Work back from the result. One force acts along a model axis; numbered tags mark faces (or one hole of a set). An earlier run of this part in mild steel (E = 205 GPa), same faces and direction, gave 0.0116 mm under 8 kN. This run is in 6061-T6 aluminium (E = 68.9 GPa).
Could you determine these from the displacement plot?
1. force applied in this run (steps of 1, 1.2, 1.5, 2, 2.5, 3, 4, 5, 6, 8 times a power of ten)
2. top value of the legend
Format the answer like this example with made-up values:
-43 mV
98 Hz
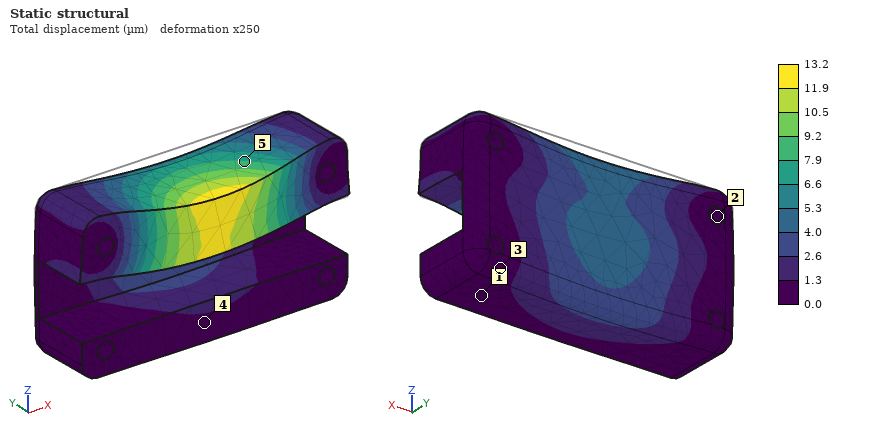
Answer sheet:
3 kN
13.2 µm
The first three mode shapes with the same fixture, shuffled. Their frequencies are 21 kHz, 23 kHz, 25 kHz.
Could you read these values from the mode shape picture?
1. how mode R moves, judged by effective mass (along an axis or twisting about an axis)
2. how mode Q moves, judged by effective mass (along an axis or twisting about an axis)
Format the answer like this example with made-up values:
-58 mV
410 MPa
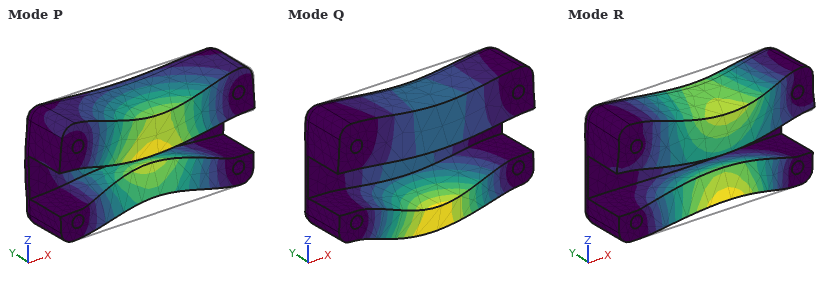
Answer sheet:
along Y
along Z
